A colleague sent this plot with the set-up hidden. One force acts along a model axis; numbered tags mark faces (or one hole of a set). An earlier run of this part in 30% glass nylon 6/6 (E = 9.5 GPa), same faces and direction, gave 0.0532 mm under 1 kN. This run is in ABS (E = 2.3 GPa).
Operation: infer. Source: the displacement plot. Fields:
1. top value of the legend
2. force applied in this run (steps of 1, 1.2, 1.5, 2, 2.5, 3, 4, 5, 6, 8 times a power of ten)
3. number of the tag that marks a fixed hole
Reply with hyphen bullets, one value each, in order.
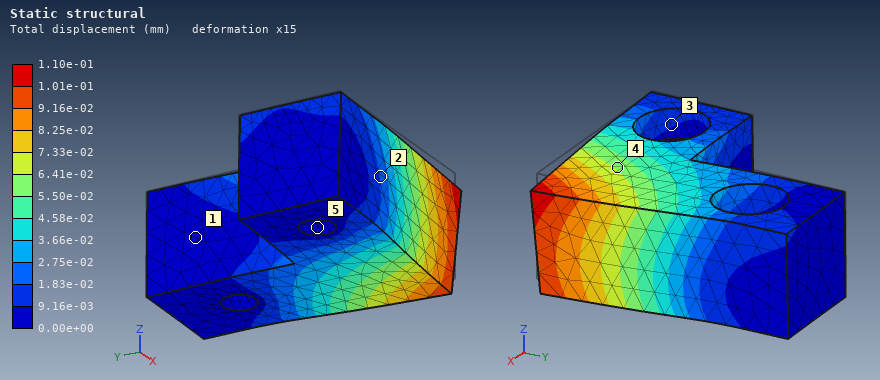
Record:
- 1.10e-01 mm
- 500 N
- 5
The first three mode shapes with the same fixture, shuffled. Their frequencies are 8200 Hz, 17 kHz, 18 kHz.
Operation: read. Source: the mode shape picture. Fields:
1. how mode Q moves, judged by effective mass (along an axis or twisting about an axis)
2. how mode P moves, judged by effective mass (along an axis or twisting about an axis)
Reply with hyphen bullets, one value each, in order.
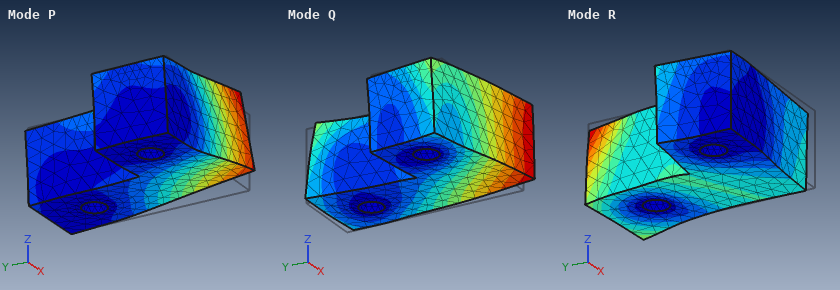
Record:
- along Y
- along Z
